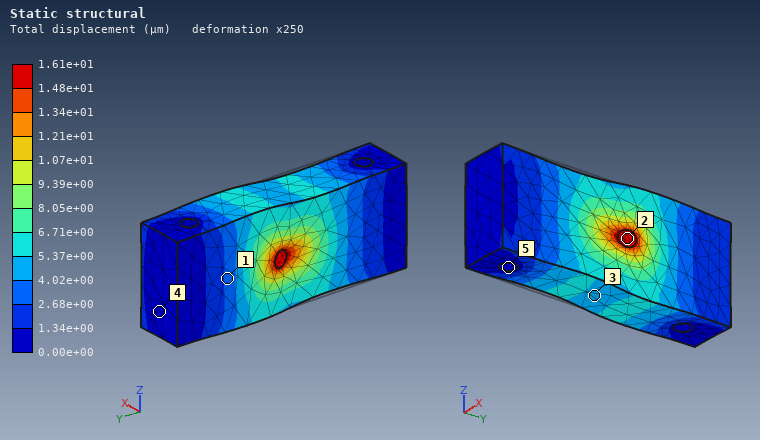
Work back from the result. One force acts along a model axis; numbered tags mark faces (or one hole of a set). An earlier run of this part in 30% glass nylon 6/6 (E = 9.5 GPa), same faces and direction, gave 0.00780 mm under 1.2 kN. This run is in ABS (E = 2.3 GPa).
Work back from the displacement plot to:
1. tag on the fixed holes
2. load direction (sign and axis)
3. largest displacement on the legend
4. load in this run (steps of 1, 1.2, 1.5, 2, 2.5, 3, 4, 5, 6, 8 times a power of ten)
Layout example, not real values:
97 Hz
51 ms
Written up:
5
+Y
1.61e+01 µm
600 N
